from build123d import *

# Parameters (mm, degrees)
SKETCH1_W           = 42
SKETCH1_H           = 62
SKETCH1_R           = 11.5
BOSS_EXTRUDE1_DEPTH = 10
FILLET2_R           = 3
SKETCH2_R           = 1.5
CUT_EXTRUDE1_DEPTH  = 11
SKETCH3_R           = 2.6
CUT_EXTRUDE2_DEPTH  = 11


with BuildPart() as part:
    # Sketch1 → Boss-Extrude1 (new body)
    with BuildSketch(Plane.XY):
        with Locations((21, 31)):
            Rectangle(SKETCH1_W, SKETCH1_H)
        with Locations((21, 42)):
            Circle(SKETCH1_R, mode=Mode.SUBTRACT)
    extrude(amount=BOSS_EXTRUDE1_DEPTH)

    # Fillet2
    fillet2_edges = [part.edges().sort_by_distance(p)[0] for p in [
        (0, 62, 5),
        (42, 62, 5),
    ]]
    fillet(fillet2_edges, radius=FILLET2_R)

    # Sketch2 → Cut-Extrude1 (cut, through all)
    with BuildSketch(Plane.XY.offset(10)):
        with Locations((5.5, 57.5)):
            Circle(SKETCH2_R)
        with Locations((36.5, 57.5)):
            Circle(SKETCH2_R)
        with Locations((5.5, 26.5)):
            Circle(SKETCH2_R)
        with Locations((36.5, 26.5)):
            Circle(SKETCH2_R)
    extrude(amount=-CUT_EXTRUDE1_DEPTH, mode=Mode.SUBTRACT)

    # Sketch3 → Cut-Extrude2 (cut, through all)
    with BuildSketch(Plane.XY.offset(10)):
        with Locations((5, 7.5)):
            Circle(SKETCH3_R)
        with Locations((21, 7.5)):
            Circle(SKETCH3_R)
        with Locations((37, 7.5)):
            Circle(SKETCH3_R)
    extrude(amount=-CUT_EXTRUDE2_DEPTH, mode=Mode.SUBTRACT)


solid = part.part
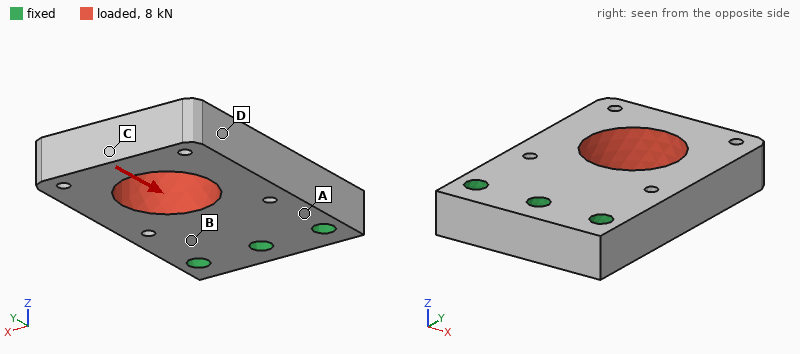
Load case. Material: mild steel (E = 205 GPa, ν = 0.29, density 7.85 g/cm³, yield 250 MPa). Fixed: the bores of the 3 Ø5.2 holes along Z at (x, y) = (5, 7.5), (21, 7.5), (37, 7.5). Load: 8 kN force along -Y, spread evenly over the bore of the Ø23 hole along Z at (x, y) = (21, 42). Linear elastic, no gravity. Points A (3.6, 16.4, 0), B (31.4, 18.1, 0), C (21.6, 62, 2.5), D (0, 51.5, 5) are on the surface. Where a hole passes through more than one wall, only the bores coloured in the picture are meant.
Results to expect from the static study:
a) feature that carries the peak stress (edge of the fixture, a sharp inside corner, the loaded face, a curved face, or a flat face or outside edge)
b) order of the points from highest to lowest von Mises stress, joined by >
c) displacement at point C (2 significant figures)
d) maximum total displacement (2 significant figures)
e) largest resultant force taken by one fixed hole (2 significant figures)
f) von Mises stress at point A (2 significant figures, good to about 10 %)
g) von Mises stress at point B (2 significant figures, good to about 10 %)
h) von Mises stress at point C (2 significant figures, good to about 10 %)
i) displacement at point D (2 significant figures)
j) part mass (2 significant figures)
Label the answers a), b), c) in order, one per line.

a) a curved face
b) C > A > B > D
c) 8.9 µm
d) 9.3 µm
e) 2.8 kN
f) 26 MPa
g) 17 MPa
h) 42 MPa
i) 3.8 µm
j) 160 g
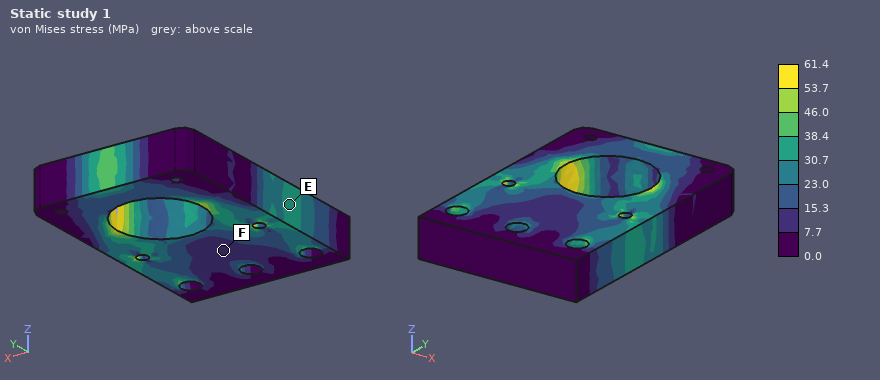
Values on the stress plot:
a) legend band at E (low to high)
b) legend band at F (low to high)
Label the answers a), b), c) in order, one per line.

a) 30.7 to 38.4 MPa
b) 7.7 to 15.3 MPa
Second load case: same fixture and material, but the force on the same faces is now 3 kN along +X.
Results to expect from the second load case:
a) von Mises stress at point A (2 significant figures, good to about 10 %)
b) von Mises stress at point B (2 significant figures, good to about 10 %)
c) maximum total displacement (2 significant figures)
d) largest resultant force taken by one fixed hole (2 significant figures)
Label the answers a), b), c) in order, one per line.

a) 24 MPa
b) 16 MPa
c) 18 µm
d) 3.1 kN
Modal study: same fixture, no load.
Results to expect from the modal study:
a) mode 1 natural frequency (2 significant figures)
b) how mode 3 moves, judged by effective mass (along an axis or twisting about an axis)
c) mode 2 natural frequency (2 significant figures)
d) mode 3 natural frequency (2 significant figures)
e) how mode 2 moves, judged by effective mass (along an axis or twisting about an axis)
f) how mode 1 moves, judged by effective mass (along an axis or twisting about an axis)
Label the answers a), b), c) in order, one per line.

a) 2900 Hz
b) along X
c) 6500 Hz
d) 7600 Hz
e) twisting about Y
f) along Z
